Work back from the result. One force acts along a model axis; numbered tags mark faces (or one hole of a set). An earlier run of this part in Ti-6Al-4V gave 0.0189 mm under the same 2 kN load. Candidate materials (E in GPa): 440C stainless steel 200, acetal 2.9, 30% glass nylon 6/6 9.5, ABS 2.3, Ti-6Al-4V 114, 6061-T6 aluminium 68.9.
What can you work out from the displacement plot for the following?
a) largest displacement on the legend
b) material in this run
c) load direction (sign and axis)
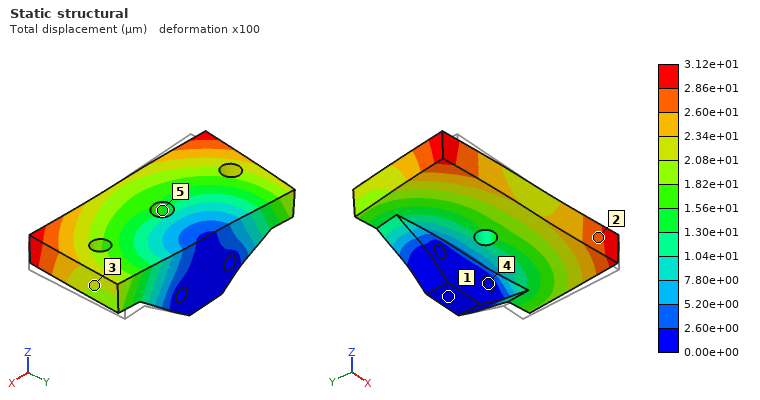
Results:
3.12e+01 µm
6061-T6 aluminium
-X
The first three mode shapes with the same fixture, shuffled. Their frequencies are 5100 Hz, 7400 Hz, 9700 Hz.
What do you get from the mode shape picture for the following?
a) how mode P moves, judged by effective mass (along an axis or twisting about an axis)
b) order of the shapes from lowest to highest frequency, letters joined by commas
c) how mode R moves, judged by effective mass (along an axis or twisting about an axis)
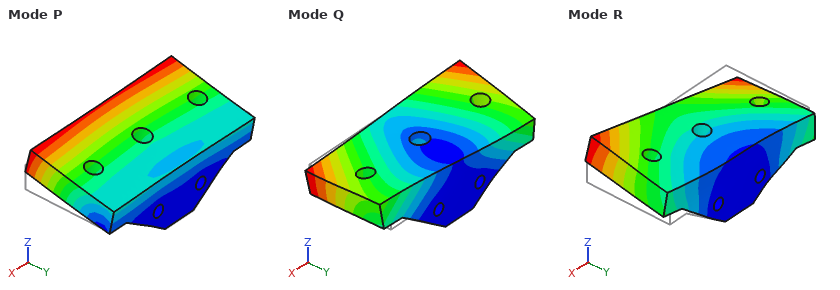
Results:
along Z
P, Q, R
along X
